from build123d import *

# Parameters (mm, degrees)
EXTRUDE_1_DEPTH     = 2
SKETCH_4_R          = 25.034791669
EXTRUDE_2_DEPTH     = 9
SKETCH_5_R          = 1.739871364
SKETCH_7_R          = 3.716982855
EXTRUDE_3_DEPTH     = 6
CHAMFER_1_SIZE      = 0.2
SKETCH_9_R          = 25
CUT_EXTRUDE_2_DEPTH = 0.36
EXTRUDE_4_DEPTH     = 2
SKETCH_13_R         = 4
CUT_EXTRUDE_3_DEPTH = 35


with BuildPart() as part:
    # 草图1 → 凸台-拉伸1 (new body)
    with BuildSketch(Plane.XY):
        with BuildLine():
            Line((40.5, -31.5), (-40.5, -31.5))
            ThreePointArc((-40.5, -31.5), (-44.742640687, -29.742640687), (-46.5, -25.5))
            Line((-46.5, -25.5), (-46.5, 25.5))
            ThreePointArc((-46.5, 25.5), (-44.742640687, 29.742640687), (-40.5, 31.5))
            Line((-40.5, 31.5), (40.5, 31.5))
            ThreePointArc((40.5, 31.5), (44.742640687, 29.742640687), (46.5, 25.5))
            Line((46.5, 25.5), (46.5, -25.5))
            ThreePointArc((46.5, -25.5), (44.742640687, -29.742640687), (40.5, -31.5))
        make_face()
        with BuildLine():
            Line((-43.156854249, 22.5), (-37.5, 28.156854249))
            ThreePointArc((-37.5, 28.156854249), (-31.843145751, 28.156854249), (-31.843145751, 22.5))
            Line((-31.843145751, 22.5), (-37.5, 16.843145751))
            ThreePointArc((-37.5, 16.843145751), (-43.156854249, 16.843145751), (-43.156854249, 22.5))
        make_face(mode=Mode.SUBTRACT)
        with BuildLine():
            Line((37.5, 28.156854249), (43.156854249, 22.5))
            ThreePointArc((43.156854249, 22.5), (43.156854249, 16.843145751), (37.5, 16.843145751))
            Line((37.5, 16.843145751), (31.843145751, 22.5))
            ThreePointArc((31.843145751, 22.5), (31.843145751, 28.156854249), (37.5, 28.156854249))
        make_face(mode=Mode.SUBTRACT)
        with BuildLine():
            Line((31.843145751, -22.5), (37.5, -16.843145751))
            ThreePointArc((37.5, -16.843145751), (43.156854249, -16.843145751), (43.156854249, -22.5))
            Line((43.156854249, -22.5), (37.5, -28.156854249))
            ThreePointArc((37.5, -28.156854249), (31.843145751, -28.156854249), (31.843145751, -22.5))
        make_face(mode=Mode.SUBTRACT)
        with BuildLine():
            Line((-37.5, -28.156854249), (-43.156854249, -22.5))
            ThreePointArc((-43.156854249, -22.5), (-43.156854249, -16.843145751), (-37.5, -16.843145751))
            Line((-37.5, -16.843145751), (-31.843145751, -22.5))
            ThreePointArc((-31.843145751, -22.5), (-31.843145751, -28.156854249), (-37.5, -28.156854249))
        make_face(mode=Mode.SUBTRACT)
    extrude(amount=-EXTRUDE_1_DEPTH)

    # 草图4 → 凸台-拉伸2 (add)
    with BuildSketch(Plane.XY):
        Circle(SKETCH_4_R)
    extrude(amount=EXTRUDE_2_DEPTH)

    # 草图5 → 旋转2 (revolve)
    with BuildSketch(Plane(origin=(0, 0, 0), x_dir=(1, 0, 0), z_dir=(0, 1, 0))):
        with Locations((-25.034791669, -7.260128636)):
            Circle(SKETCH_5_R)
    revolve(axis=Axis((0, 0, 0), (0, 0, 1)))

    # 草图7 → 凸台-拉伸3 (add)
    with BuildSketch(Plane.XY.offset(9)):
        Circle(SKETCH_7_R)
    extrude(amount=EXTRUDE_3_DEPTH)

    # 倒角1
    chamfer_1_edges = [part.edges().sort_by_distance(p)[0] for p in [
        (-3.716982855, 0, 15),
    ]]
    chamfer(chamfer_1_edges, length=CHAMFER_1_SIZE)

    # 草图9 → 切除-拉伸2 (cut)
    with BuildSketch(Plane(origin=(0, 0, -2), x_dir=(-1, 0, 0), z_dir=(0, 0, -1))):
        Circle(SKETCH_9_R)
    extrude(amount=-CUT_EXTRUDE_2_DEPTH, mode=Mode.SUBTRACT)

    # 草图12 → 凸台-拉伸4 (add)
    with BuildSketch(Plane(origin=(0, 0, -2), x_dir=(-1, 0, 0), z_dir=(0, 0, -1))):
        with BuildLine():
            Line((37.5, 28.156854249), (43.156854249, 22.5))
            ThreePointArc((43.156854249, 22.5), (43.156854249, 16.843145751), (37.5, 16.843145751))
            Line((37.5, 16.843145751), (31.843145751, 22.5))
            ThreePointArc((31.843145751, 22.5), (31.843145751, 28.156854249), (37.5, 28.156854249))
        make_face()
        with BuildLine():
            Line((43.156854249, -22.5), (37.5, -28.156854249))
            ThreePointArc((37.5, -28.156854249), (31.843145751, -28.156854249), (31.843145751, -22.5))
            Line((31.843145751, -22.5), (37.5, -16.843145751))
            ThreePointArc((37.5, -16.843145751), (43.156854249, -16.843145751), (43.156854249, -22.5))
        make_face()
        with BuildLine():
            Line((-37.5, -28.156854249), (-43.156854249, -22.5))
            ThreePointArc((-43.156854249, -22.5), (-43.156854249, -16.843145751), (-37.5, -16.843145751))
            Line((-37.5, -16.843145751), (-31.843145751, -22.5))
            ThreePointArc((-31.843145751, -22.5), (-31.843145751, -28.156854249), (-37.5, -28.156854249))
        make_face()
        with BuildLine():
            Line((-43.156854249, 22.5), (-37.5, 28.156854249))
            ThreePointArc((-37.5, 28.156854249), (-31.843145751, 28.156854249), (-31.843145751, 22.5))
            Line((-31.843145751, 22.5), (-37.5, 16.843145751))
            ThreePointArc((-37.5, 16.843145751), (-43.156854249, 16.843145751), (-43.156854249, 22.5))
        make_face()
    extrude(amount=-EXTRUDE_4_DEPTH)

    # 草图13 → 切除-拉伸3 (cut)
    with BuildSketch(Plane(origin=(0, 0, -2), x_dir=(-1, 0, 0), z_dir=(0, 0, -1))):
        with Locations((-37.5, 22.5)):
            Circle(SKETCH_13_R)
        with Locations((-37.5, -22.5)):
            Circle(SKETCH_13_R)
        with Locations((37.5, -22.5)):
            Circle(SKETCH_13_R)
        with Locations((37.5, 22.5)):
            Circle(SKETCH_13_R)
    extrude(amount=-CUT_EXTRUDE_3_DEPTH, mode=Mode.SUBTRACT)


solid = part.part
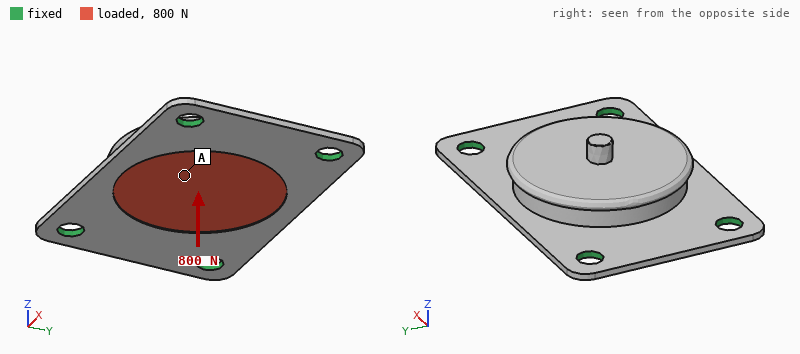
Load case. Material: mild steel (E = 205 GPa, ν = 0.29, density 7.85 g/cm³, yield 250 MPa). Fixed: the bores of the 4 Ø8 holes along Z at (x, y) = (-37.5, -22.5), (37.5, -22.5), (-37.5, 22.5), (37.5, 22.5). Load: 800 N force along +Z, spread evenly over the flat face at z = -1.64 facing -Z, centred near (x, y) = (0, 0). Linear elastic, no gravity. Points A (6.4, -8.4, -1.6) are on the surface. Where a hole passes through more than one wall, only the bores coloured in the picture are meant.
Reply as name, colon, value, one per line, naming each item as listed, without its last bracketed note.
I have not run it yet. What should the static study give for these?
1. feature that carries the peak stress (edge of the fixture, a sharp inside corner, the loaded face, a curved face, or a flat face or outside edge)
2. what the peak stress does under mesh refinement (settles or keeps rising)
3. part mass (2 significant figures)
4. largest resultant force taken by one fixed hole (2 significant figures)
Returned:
feature that carries the peak stress: edge of the fixture
what the peak stress does under mesh refinement: keeps rising
part mass: 230 g
largest resultant force taken by one fixed hole: 290 N
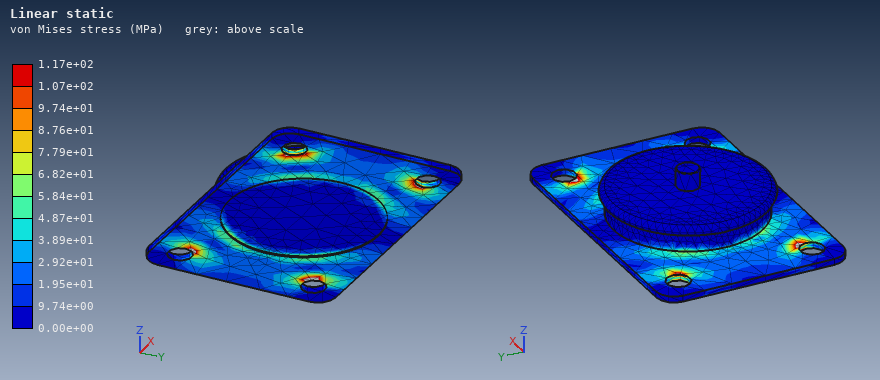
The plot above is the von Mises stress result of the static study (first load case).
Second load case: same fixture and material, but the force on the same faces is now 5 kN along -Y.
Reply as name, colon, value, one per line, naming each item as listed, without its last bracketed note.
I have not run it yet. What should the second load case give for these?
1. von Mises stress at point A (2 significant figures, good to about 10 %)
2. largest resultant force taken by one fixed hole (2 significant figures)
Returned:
von Mises stress at point A: 8.1 MPa
largest resultant force taken by one fixed hole: 1.4 kN
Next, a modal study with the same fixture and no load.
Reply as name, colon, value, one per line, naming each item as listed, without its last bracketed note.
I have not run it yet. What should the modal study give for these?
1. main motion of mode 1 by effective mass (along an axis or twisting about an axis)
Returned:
main motion of mode 1 by effective mass: along Z
